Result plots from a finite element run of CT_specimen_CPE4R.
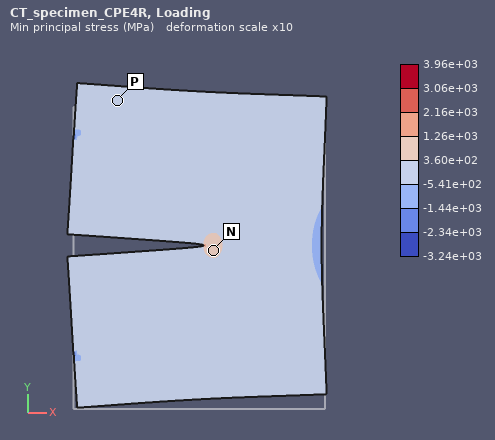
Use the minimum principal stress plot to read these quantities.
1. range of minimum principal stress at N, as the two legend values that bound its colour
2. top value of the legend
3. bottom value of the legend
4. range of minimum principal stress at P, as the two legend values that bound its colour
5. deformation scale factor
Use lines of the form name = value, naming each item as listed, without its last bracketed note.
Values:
range of minimum principal stress at N, as the two legend values that bound its colour = 3.60e+02 to 1.26e+03 MPa
top value of the legend = 3.96e+03 MPa
bottom value of the legend = -3.24e+03 MPa
range of minimum principal stress at P, as the two legend values that bound its colour = -5.41e+02 to 3.60e+02 MPa
deformation scale factor = 10
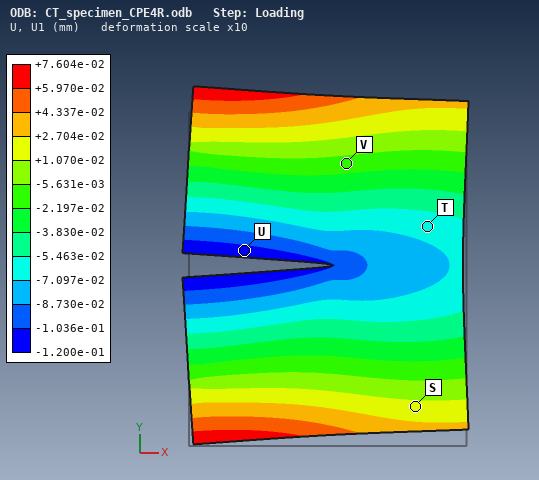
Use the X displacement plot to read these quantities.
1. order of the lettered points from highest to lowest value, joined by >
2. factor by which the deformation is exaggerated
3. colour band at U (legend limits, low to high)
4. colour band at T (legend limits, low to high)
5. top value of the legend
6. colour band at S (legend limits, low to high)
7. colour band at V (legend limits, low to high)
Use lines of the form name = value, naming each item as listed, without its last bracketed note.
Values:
order of the lettered points from highest to lowest value, joined by > = S > V > T > U
factor by which the deformation is exaggerated = 10
colour band at U = -1.200e-01 to -1.036e-01 mm
colour band at T = -7.097e-02 to -5.463e-02 mm
top value of the legend = +7.604e-02 mm
colour band at S = +1.070e-02 to +2.704e-02 mm
colour band at V = -2.197e-02 to -5.631e-03 mm
